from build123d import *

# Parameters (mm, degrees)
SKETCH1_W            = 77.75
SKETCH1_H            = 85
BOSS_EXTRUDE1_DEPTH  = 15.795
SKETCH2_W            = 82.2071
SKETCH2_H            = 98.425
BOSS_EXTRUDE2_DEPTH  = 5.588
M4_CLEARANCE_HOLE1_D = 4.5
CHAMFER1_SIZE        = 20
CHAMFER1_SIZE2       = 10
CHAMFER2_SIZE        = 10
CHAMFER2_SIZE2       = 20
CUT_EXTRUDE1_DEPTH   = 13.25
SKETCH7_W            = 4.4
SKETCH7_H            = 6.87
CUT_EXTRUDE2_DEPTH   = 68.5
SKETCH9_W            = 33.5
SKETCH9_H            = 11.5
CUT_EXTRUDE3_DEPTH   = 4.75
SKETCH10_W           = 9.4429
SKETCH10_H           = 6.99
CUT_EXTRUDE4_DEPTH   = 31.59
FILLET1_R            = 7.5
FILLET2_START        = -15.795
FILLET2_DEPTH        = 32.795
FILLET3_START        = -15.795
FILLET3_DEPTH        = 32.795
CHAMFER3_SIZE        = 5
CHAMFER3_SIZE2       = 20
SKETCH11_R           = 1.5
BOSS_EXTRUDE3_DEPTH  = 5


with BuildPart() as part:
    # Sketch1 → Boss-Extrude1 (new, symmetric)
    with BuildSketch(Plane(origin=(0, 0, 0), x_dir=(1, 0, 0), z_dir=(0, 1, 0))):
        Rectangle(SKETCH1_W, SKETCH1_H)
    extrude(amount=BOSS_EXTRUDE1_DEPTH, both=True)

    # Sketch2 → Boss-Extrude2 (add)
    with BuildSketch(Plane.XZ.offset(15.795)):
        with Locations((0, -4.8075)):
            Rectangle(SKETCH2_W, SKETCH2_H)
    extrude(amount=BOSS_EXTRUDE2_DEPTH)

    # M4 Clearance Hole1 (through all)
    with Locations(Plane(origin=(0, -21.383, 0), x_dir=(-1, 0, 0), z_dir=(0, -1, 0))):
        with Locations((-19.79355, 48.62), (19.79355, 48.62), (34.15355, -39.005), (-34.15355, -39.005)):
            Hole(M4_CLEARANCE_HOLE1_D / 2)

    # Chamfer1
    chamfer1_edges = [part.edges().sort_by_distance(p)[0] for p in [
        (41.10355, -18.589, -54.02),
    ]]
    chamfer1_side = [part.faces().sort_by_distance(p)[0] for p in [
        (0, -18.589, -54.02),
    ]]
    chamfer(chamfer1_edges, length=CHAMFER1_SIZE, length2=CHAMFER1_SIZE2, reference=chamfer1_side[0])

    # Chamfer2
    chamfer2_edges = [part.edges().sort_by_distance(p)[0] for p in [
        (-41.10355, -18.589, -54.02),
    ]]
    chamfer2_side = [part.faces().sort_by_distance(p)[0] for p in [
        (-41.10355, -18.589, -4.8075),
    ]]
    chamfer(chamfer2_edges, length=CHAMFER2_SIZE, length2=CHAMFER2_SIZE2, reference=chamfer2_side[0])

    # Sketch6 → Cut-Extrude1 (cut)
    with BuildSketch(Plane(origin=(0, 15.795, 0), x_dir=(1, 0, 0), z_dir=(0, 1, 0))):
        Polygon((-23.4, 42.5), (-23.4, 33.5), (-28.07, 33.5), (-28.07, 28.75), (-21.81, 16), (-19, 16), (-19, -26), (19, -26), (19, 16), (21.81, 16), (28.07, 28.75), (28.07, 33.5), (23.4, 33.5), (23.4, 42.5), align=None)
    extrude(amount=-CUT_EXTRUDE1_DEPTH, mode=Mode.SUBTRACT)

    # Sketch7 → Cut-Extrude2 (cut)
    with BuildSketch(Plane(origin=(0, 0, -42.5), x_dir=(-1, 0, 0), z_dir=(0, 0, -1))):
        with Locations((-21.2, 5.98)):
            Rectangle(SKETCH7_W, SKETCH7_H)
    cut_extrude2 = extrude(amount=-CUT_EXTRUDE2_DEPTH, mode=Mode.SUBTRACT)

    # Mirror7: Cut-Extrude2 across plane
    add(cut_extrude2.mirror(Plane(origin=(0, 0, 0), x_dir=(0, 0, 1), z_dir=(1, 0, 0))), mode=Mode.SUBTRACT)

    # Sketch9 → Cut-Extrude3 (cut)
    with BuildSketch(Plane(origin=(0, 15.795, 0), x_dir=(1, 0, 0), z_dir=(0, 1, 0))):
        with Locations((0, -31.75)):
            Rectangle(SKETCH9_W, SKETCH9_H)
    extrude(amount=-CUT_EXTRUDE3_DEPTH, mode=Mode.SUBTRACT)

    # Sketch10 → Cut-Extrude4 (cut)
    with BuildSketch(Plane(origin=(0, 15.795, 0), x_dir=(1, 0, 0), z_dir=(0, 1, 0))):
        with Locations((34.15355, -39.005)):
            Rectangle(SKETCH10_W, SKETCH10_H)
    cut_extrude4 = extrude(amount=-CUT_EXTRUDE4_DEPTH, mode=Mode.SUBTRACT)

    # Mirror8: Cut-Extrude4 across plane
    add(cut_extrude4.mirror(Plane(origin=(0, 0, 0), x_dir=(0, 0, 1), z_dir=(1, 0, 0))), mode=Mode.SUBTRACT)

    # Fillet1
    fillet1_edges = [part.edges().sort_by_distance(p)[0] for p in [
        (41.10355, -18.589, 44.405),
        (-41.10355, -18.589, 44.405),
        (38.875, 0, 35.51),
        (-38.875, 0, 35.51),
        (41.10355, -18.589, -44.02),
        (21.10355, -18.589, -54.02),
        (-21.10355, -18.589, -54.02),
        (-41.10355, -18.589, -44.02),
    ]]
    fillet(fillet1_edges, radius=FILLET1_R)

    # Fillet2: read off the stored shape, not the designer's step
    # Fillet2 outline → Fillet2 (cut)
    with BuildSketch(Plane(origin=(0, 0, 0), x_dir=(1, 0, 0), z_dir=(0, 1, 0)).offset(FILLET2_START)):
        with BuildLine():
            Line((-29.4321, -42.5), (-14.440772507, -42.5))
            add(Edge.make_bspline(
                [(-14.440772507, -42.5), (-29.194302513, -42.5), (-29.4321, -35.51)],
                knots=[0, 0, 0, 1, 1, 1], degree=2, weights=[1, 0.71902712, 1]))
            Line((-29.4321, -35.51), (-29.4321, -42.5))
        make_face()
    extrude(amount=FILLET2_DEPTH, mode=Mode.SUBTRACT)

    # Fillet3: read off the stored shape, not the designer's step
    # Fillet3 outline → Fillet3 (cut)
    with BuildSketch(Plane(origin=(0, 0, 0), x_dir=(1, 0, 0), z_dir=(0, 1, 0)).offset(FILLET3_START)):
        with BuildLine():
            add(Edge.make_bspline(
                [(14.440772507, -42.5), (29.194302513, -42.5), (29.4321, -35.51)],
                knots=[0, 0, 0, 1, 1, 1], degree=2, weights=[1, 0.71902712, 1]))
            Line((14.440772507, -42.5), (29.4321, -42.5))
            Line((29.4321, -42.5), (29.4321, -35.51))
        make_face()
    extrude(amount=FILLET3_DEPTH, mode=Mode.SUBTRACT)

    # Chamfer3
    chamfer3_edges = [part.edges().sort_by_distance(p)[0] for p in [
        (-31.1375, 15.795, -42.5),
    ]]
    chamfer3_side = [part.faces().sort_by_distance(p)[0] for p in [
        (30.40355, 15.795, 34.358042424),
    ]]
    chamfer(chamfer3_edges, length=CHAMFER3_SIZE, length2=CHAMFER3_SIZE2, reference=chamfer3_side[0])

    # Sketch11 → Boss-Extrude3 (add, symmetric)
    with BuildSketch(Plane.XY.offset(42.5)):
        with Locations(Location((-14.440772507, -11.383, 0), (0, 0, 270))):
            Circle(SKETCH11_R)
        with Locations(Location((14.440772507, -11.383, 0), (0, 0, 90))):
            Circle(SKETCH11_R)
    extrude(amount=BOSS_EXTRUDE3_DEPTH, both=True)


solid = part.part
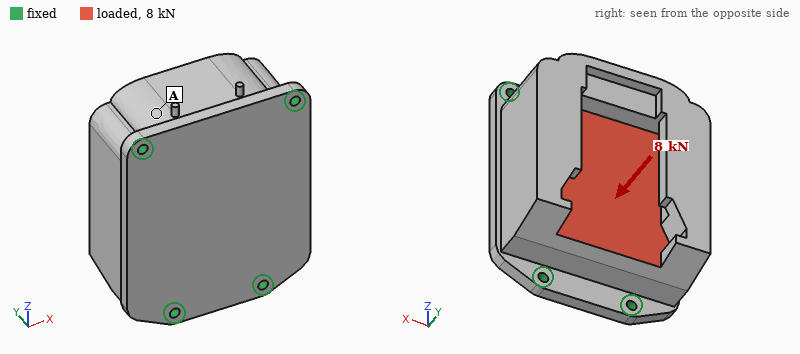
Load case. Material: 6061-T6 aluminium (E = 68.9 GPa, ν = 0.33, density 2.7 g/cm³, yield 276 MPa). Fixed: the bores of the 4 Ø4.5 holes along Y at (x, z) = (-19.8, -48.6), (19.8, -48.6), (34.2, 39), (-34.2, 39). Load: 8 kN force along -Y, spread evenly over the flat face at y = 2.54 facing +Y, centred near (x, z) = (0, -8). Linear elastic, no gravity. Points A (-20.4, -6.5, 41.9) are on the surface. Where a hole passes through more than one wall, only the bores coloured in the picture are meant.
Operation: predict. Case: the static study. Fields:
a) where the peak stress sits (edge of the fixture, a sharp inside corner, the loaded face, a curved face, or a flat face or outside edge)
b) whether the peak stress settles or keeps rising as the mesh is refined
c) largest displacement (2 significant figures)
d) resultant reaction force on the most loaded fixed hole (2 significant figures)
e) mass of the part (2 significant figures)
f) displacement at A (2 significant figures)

edge of the fixture
keeps rising
18 µm
2.4 kN
540 g
8.3 µm
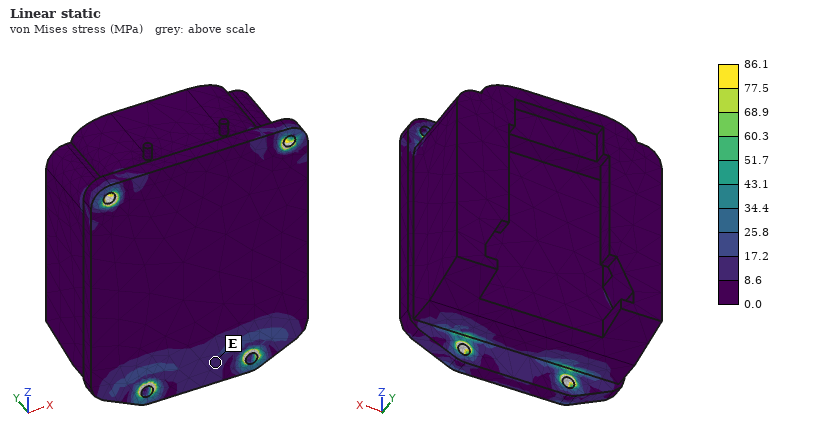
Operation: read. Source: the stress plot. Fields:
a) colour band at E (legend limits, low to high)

8.6 to 17.2 MPa
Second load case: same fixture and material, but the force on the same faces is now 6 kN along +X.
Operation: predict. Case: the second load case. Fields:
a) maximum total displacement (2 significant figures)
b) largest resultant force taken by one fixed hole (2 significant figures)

20 µm
2.4 kN
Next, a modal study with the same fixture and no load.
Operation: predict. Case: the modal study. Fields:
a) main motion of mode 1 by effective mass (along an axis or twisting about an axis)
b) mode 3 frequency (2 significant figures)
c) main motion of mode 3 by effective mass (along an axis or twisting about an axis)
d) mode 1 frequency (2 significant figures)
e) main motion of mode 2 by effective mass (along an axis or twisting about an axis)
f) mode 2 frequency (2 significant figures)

along X
7400 Hz
along Z
5000 Hz
along Y
5200 Hz
